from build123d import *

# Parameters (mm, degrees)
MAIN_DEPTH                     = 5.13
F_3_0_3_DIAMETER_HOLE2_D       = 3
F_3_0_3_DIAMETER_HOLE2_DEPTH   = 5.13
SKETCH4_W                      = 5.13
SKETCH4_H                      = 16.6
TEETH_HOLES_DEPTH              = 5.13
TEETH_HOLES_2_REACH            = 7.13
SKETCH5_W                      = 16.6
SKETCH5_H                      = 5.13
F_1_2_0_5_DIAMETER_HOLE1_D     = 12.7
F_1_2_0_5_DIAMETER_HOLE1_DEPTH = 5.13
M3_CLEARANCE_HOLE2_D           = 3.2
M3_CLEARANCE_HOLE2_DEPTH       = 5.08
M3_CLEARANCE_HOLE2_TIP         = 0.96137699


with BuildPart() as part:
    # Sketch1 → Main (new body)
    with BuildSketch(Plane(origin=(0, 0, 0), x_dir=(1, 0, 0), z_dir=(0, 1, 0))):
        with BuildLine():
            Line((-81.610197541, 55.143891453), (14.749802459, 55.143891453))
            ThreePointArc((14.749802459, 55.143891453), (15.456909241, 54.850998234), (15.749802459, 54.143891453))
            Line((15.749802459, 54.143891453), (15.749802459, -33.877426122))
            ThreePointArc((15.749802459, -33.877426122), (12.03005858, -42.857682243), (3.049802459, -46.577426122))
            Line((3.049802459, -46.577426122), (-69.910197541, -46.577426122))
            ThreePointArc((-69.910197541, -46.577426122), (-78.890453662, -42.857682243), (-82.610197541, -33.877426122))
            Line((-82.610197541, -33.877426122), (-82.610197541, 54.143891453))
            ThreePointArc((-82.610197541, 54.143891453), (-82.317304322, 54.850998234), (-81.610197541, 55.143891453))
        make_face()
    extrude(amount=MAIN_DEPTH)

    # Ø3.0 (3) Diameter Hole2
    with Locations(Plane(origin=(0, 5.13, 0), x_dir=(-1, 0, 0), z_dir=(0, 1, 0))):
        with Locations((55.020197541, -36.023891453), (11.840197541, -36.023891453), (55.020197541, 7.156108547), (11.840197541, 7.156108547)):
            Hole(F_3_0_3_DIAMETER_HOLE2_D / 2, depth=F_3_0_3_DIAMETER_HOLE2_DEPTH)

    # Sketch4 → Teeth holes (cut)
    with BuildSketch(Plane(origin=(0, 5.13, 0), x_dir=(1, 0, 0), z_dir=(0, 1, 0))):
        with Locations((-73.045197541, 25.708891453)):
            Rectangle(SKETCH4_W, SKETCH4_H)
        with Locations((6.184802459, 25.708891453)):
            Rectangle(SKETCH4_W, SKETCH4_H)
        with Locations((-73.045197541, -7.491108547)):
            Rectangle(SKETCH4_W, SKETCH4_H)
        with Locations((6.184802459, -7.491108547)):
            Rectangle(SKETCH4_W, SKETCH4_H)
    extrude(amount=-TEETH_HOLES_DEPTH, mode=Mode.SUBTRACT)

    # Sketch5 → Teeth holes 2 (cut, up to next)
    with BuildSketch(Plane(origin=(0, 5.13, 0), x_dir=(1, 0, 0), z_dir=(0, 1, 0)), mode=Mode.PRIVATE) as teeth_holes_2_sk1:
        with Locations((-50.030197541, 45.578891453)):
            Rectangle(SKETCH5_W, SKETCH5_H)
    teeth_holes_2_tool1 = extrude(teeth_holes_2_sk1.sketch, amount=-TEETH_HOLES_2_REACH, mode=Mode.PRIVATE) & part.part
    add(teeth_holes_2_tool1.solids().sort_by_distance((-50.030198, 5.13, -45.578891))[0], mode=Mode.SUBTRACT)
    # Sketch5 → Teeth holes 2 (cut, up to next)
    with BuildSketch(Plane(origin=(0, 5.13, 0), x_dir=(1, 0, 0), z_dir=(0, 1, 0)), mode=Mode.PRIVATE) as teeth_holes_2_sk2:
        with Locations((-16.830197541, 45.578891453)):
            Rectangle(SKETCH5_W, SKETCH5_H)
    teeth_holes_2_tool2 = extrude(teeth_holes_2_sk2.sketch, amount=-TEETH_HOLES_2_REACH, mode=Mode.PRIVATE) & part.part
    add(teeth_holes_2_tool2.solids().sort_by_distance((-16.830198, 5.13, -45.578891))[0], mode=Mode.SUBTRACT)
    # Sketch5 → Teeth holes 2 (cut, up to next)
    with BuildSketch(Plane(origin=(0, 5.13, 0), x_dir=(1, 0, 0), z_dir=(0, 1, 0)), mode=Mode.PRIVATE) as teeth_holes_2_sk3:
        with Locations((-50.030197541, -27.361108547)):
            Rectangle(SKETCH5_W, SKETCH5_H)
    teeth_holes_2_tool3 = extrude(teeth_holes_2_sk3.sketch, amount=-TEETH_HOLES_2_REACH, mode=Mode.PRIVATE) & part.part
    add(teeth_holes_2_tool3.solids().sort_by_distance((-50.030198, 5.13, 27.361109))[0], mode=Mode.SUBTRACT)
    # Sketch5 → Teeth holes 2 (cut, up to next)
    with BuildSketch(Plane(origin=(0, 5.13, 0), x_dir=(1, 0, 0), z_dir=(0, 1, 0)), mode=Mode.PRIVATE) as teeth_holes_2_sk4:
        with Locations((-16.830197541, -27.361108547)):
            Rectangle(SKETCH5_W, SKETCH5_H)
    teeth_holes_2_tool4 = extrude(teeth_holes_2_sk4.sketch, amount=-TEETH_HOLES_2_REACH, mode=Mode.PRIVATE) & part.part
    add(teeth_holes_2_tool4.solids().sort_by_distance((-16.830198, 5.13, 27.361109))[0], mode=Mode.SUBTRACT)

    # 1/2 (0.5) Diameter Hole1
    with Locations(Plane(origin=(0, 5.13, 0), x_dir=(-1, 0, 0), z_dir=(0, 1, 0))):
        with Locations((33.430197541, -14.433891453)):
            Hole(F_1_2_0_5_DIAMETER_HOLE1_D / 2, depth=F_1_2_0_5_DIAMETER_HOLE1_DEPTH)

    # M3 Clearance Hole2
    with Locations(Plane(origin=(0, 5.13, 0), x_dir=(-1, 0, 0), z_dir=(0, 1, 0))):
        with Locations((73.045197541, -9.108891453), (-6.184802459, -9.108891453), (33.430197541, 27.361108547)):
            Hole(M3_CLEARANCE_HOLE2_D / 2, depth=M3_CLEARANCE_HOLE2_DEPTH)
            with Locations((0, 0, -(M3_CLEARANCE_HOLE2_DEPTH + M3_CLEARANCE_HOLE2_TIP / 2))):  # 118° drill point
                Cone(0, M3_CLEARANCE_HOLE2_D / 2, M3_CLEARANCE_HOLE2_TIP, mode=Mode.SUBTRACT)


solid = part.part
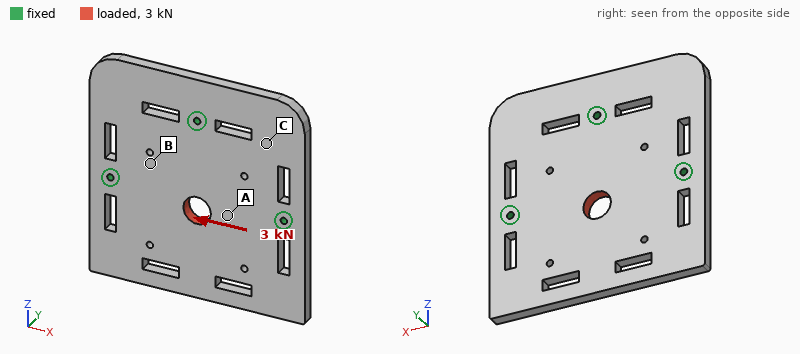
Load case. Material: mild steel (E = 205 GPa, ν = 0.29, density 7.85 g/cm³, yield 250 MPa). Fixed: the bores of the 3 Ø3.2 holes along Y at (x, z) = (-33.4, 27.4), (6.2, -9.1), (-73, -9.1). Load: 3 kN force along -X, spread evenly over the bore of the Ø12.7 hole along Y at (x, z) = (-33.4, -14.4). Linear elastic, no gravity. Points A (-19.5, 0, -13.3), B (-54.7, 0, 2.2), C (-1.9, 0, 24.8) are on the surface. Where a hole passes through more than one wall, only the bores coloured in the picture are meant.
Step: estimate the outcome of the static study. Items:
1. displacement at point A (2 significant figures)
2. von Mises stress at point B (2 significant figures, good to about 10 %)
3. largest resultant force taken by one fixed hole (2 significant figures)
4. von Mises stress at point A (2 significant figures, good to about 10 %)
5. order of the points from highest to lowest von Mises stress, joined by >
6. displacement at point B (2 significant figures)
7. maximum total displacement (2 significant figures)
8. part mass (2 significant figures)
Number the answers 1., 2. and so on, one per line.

1. 1.9 µm
2. 4.7 MPa
3. 1.3 kN
4. 14 MPa
5. A > B > C
6. 1.1 µm
7. 2.8 µm
8. 370 g
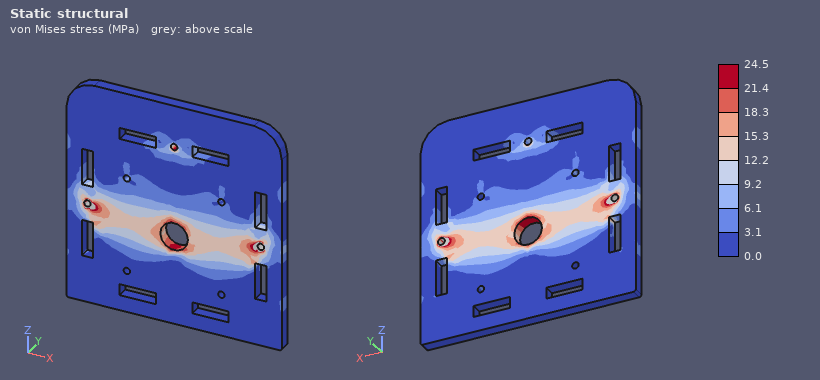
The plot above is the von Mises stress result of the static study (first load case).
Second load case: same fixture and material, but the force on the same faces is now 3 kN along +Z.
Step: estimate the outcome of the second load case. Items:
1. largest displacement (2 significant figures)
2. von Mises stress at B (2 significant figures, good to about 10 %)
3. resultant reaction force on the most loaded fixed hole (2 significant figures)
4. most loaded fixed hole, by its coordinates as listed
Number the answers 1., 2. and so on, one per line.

1. 3.1 µm
2. 5.2 MPa
3. 1.3 kN
4. (-33.4, 27.4)
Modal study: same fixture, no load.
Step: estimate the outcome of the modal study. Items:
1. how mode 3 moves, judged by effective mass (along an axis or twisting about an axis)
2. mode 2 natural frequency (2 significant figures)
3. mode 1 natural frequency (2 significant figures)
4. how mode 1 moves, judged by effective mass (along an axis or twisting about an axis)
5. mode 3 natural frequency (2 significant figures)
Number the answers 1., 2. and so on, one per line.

1. twisting about Z
2. 2500 Hz
3. 1400 Hz
4. along Y
5. 2700 Hz
